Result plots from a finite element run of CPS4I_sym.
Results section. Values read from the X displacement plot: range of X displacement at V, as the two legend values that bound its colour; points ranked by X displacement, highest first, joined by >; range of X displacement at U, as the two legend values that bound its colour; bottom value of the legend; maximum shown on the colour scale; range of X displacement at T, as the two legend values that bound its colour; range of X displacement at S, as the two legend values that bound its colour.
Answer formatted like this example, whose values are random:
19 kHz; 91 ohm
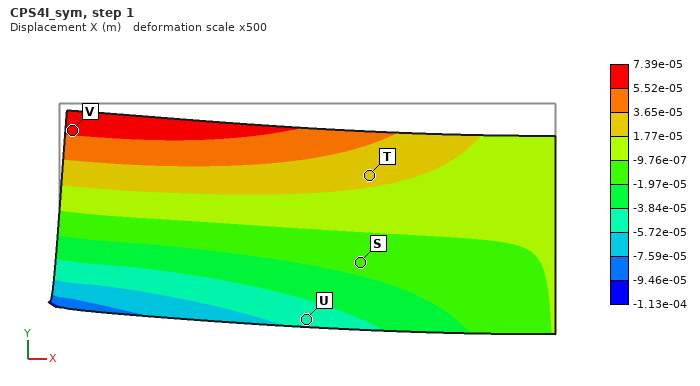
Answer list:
5.52e-05 to 7.39e-05 m; V > T > S > U; -5.72e-05 to -3.84e-05 m; -1.13e-04 m; 7.39e-05 m; 1.77e-05 to 3.65e-05 m; -1.97e-05 to -9.76e-07 m
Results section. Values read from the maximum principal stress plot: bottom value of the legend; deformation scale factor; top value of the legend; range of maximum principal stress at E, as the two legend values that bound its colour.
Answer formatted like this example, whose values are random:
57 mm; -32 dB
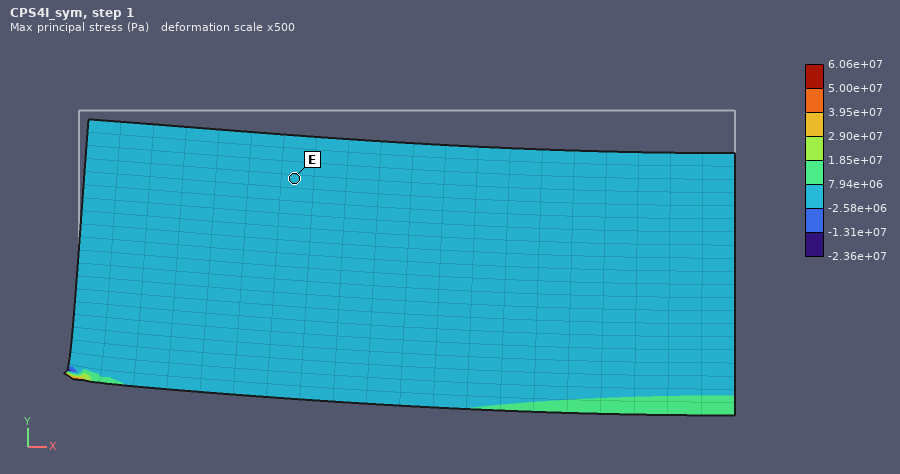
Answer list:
-2.36e+07 Pa; 500; 6.06e+07 Pa; -2.58e+06 to 7.94e+06 Pa
